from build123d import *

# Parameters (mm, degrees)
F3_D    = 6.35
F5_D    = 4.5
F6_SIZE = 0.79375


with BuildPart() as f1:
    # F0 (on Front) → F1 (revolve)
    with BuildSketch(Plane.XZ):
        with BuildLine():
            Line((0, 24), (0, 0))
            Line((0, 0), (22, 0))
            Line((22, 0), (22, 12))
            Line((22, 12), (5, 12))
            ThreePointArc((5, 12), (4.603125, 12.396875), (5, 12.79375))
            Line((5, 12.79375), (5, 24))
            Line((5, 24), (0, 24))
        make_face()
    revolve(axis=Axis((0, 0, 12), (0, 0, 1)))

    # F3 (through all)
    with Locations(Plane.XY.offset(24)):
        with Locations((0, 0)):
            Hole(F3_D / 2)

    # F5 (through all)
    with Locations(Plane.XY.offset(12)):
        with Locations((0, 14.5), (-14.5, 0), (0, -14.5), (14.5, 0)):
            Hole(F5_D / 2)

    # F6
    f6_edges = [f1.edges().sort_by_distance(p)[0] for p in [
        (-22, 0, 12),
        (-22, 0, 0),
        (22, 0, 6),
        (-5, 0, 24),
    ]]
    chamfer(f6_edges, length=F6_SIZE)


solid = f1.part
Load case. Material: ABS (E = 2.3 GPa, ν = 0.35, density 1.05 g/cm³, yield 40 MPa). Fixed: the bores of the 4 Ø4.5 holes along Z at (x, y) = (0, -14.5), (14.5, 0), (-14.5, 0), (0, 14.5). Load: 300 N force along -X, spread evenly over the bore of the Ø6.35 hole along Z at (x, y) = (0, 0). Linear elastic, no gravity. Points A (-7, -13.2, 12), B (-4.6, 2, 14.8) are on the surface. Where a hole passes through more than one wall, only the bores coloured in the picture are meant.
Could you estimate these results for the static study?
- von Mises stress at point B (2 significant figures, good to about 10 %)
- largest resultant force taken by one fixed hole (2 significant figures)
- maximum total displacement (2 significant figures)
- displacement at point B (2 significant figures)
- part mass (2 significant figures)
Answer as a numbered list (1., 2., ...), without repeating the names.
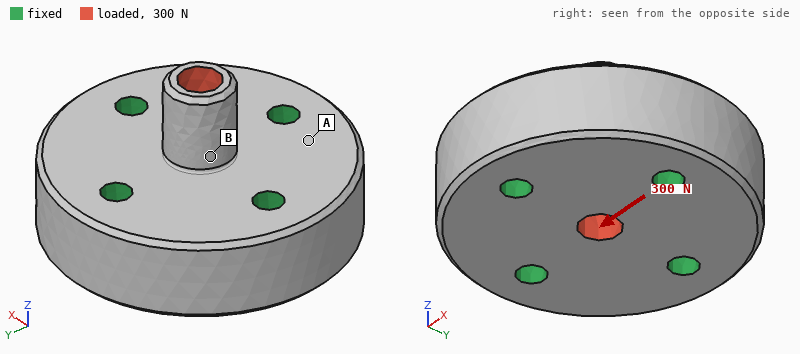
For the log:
1. 4.8 MPa
2. 120 N
3. 0.13 mm
4. 0.051 mm
5. 18 g
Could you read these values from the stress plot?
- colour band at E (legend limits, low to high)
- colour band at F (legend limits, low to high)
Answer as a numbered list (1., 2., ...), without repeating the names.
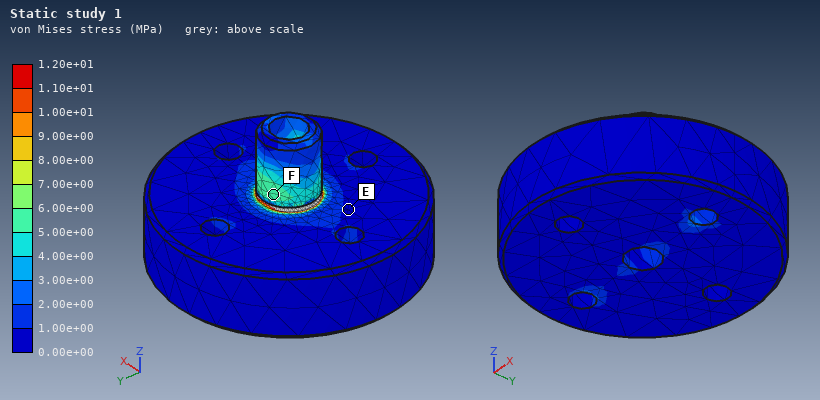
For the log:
1. 0.00e+00 to 1.00e+00 MPa
2. 5.00e+00 to 6.00e+00 MPa
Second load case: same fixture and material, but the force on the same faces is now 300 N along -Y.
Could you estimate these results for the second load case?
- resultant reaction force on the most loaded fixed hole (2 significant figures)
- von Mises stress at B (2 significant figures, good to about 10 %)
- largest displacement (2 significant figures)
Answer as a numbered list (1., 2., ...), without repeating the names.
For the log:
1. 120 N
2. 5.8 MPa
3. 0.13 mm
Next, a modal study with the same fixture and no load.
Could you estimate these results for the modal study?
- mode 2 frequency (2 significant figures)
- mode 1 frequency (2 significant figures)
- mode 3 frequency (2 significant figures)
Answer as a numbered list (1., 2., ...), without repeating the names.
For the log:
1. 8300 Hz
2. 8300 Hz
3. 14 kHz
